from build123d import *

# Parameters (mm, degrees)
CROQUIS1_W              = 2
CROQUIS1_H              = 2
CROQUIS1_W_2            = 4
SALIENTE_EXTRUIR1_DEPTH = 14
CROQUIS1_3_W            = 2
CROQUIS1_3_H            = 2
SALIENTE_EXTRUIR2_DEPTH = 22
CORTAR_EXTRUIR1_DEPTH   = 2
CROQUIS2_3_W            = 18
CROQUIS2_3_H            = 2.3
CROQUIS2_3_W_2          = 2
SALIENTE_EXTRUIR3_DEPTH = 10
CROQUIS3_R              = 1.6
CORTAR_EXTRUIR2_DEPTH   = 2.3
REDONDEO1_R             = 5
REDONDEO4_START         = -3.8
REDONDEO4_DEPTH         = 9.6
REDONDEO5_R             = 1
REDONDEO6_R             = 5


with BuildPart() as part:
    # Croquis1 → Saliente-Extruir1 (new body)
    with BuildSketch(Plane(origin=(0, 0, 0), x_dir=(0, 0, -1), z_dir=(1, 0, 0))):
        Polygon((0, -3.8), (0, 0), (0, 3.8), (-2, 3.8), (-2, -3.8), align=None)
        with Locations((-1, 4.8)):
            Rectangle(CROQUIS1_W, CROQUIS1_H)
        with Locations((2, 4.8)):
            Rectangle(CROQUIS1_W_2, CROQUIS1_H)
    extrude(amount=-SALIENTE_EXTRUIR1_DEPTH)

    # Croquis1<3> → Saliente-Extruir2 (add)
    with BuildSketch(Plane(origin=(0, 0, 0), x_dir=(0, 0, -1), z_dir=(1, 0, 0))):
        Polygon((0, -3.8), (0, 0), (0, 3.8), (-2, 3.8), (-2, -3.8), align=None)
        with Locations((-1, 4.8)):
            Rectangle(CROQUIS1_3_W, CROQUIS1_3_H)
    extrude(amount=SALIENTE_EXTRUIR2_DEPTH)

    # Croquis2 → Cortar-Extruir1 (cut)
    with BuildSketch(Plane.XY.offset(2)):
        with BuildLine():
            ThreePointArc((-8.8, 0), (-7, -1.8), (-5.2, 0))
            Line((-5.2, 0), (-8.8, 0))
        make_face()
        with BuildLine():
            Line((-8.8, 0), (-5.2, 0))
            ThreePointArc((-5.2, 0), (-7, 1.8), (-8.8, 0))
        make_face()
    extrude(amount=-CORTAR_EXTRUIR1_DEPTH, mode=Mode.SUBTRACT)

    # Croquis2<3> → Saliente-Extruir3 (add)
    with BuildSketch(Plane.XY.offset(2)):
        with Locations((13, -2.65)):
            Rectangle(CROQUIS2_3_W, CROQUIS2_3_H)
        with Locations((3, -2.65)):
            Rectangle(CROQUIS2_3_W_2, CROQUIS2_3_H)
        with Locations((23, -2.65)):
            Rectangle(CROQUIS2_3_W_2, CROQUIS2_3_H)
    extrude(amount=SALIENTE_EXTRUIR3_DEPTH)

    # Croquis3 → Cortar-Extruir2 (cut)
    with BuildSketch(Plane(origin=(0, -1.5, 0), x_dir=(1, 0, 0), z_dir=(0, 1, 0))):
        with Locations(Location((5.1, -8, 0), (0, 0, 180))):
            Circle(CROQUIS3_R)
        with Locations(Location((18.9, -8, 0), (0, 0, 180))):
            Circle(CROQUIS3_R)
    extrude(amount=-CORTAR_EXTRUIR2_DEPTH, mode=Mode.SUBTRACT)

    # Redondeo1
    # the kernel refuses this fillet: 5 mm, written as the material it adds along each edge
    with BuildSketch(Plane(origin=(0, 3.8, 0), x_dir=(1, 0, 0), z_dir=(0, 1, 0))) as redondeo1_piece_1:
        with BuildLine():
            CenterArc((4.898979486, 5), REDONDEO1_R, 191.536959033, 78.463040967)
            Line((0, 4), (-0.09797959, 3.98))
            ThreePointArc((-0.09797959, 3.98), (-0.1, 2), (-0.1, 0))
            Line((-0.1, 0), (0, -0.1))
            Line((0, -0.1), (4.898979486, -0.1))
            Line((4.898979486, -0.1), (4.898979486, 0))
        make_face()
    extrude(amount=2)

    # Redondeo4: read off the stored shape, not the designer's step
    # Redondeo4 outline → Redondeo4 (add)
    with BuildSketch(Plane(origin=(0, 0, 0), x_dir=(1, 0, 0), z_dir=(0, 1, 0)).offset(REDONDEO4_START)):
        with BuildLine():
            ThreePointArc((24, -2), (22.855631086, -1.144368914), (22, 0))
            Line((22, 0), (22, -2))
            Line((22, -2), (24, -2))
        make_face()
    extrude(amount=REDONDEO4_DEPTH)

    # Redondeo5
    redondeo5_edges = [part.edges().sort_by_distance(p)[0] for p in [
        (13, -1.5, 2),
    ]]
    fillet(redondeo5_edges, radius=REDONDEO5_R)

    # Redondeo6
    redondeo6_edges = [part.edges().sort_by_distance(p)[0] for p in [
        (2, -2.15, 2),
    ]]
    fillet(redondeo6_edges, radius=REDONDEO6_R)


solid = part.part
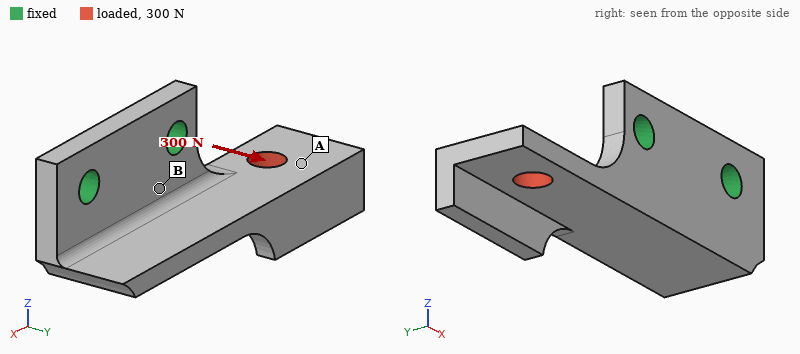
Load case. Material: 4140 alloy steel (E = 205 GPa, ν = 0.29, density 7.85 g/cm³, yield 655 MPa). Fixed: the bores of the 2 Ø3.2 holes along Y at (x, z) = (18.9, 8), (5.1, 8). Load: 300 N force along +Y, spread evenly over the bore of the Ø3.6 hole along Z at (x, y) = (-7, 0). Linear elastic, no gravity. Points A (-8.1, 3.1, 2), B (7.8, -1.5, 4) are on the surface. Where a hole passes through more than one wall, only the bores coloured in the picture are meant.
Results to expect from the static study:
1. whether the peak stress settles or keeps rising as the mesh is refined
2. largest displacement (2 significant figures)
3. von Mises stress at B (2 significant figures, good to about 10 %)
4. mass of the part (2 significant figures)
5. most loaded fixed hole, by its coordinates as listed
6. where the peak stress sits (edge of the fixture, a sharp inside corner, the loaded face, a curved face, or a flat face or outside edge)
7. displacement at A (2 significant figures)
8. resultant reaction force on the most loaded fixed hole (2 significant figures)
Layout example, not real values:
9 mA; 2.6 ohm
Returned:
keeps rising; 89 µm; 110 MPa; 10 g; (5.1, 8); edge of the fixture; 54 µm; 510 N
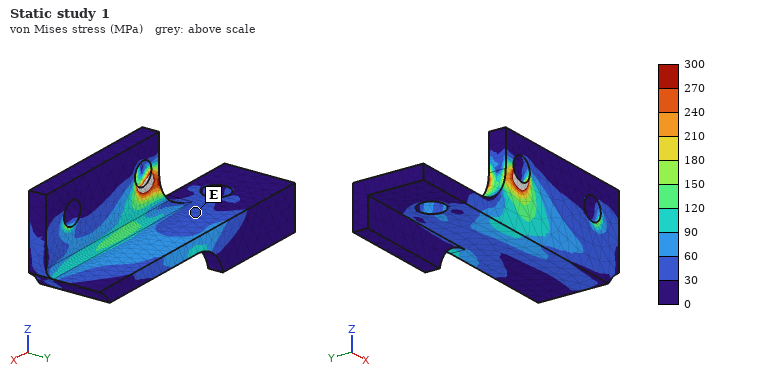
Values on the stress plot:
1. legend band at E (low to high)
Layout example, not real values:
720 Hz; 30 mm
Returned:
30 to 60 MPa
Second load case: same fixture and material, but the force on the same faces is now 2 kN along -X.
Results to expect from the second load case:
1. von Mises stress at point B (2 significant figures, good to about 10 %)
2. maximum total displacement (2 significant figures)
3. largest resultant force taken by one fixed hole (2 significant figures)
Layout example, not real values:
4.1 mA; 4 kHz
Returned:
170 MPa; 36 µm; 1.3 kN
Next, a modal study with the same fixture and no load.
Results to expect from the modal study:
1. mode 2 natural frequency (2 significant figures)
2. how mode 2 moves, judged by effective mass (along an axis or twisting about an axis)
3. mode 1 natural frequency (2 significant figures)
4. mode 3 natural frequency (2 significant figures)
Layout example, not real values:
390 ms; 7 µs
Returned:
7700 Hz; along Y; 4400 Hz; 12 kHz
